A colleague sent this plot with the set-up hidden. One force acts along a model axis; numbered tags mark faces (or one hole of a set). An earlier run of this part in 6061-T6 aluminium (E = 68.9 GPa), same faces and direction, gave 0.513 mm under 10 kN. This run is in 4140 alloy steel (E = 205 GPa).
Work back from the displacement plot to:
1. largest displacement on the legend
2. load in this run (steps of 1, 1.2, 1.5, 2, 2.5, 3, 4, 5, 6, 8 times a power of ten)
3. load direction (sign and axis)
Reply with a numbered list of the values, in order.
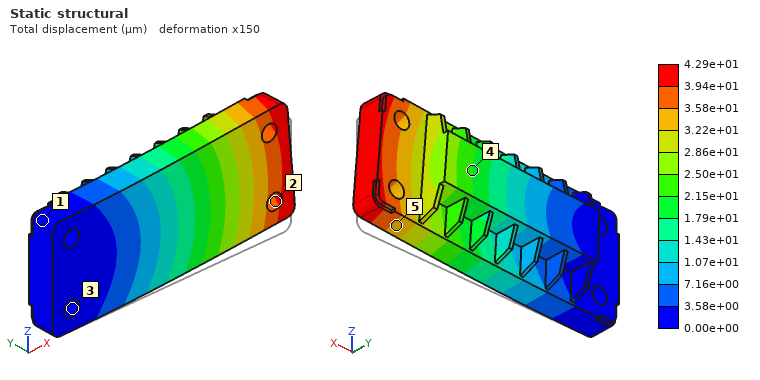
1. 4.29e+01 µm
2. 2.5 kN
3. +Z
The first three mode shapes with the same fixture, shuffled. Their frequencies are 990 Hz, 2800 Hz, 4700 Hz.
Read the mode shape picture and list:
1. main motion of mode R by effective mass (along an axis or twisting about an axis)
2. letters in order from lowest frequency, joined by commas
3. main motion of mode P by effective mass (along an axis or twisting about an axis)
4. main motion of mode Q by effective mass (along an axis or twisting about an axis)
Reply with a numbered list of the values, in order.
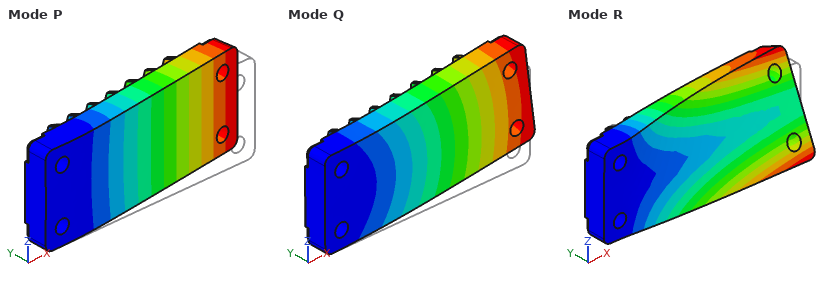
1. twisting about X
2. P, Q, R
3. along Y
4. along Z
